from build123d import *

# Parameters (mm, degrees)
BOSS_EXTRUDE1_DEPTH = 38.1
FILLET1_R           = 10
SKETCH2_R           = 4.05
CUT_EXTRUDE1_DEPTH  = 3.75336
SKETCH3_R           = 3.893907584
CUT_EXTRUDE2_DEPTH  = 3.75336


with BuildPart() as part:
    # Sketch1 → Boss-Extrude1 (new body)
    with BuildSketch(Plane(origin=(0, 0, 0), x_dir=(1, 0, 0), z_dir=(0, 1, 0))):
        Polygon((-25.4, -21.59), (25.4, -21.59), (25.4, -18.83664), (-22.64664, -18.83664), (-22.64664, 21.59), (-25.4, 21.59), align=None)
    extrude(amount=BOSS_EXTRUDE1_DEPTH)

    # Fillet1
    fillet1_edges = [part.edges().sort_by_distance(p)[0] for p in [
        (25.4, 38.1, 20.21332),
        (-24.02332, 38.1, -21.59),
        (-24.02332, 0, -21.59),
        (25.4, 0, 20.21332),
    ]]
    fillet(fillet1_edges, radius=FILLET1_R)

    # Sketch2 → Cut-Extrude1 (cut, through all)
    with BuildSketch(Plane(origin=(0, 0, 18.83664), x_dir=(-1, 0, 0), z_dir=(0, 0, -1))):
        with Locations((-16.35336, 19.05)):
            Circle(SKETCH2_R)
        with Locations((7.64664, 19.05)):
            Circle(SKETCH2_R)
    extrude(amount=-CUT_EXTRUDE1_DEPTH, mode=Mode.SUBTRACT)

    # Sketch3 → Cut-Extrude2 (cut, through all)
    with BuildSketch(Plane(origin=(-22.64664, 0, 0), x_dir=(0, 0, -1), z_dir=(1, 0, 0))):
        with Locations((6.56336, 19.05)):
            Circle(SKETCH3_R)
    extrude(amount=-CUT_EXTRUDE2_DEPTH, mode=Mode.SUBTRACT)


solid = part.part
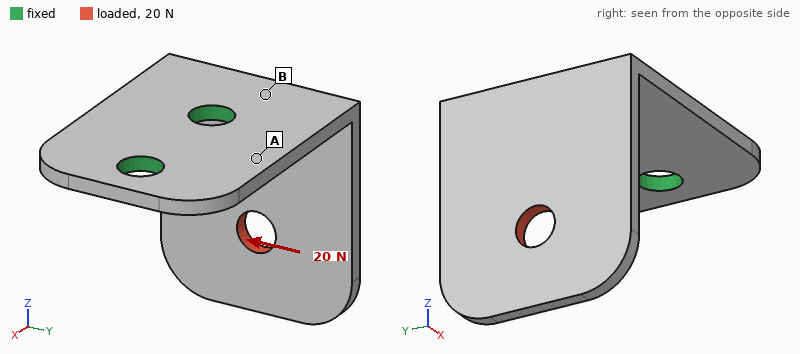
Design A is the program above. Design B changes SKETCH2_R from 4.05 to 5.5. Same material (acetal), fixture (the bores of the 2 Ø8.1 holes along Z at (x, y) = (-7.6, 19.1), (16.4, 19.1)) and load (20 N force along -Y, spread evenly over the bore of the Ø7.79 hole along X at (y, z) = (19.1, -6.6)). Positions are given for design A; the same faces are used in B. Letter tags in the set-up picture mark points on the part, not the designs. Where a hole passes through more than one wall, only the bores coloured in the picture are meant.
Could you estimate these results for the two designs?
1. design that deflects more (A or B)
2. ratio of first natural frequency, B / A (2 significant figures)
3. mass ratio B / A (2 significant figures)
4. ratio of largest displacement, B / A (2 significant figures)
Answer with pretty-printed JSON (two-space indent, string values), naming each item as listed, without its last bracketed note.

{
  "design that deflects more": "A",
  "ratio of first natural frequency, B / A": "1.0",
  "mass ratio B / A": "0.97",
  "ratio of largest displacement, B / A": "0.79"
}
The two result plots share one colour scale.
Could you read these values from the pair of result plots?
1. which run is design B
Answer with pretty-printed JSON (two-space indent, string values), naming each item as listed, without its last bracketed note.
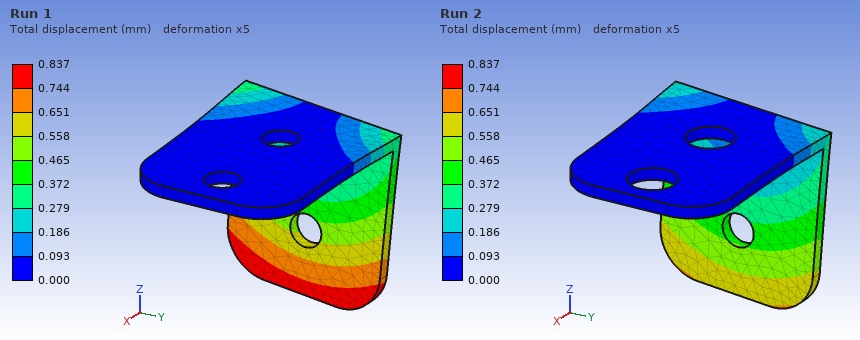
{
  "which run is design B": "Run 2"
}
